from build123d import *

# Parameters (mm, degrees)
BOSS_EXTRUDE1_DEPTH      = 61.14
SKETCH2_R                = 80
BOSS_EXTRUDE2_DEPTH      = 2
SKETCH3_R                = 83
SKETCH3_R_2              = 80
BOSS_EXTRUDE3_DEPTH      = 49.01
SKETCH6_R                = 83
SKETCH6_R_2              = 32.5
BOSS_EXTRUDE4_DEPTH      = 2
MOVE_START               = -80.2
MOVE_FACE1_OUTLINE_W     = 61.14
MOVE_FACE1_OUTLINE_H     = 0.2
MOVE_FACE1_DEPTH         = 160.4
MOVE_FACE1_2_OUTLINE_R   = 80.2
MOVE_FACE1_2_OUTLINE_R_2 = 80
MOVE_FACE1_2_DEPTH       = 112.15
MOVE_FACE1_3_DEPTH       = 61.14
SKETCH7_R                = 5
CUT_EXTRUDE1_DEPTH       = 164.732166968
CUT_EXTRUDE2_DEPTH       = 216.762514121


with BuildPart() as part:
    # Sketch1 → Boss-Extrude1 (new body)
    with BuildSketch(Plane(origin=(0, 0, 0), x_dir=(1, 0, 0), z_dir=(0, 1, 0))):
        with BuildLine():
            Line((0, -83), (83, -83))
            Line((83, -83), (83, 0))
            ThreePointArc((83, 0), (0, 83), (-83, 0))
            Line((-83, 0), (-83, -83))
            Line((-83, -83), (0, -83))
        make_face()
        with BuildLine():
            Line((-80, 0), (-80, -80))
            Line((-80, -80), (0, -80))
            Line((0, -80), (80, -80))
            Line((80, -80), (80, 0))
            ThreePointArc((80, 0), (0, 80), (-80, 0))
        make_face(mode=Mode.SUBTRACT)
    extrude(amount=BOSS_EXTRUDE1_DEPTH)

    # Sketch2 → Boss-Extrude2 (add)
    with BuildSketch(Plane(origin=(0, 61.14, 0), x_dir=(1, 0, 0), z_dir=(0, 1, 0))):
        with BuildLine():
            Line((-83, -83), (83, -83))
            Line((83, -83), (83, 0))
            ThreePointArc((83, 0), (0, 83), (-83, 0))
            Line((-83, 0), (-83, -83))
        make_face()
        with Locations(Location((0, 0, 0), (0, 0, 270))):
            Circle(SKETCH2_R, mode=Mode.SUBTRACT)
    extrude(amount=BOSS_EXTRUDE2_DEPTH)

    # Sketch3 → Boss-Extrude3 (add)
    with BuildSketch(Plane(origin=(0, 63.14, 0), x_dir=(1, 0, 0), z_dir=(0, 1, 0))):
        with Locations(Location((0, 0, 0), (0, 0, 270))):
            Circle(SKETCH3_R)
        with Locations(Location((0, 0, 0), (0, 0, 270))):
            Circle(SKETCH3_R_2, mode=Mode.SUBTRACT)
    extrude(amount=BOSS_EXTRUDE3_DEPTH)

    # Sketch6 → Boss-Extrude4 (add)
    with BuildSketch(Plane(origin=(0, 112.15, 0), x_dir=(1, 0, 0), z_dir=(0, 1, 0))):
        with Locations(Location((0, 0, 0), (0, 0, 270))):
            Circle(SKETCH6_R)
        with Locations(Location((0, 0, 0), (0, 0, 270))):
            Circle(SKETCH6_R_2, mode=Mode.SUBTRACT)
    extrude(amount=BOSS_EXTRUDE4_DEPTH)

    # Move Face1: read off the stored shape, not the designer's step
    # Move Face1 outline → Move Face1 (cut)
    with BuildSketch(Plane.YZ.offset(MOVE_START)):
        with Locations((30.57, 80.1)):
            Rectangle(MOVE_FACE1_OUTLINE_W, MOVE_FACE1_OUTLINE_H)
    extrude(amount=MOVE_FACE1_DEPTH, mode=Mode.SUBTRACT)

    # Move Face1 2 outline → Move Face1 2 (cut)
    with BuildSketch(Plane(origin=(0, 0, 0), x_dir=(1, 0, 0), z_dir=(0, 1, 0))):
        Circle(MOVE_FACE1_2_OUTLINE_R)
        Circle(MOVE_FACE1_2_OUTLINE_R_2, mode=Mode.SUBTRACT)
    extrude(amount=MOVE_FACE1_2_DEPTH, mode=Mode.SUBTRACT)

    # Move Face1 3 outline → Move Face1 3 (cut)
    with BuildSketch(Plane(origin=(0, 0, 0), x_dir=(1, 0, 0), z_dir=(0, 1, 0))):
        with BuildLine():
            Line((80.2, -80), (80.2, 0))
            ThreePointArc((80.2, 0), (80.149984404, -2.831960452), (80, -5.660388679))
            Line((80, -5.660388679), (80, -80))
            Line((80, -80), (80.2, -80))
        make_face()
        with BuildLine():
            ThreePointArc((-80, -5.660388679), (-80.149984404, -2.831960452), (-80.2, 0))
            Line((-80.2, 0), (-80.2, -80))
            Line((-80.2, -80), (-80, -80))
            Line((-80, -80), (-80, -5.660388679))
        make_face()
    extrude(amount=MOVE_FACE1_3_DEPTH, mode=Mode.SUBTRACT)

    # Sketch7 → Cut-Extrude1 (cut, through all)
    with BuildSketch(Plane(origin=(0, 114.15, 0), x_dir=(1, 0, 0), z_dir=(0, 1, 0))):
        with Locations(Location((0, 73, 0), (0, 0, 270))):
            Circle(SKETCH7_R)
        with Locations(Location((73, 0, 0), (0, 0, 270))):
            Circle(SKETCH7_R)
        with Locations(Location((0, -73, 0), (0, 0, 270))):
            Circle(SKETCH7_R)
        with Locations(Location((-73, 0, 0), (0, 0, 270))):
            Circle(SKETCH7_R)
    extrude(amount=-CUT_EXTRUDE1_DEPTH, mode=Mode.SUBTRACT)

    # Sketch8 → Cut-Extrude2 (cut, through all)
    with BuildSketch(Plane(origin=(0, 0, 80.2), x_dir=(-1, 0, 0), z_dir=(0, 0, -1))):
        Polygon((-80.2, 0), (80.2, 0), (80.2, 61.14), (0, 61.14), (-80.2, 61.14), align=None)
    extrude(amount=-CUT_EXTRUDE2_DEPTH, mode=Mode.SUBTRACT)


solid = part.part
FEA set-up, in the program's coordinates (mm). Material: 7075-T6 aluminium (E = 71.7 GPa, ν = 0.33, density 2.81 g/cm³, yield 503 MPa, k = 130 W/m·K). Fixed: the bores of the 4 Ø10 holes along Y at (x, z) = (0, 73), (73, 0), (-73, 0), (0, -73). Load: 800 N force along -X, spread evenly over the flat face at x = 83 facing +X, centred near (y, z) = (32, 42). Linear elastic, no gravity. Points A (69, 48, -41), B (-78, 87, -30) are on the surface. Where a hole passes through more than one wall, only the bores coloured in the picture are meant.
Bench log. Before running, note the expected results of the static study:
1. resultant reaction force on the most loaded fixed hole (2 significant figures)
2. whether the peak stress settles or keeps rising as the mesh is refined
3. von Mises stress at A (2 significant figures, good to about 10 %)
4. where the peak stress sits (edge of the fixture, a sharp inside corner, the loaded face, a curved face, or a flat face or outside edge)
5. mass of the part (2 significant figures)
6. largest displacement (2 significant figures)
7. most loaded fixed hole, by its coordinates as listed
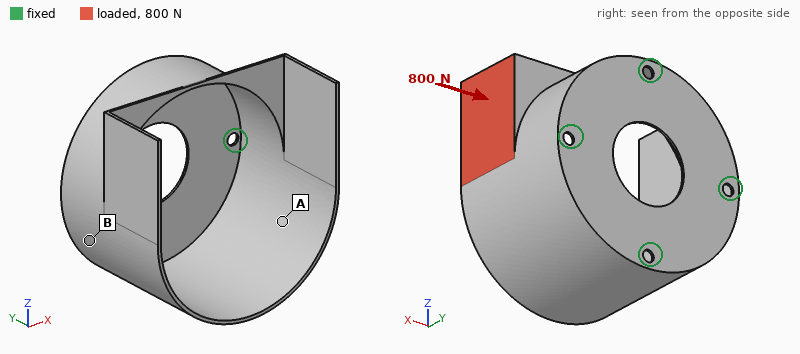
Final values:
1.1 kN
keeps rising
28 MPa
edge of the fixture
530 g
2.7 mm
(73, 0)
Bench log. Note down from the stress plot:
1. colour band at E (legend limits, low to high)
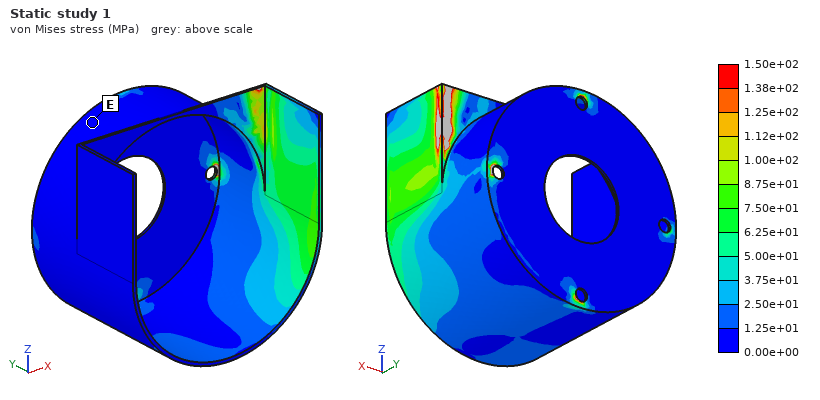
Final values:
0.00e+00 to 1.25e+01 MPa
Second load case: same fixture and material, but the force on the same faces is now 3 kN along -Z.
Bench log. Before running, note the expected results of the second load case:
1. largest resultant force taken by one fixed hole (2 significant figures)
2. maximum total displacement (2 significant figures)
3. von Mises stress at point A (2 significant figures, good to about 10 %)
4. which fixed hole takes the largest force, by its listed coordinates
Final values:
2.3 kN
2.6 mm
91 MPa
(73, 0)
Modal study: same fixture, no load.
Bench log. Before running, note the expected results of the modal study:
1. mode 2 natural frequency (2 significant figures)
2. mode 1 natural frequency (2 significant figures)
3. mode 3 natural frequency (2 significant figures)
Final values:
600 Hz
390 Hz
640 Hz
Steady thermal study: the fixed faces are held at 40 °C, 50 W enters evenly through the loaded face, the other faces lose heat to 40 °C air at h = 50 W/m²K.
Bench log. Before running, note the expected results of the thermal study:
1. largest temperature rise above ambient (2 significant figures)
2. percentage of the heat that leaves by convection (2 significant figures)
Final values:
60 K
81 %
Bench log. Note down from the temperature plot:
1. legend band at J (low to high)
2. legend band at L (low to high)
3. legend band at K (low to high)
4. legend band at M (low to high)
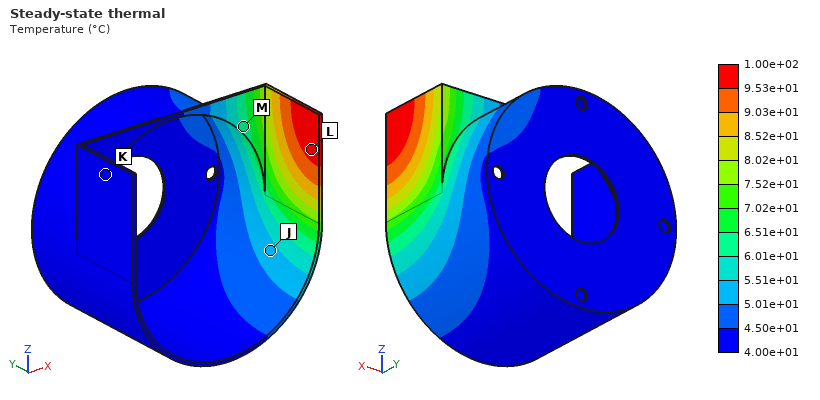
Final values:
5.01e+01 to 5.51e+01 °C
9.53e+01 to 1.00e+02 °C
4.00e+01 to 4.50e+01 °C
6.01e+01 to 6.51e+01 °C
